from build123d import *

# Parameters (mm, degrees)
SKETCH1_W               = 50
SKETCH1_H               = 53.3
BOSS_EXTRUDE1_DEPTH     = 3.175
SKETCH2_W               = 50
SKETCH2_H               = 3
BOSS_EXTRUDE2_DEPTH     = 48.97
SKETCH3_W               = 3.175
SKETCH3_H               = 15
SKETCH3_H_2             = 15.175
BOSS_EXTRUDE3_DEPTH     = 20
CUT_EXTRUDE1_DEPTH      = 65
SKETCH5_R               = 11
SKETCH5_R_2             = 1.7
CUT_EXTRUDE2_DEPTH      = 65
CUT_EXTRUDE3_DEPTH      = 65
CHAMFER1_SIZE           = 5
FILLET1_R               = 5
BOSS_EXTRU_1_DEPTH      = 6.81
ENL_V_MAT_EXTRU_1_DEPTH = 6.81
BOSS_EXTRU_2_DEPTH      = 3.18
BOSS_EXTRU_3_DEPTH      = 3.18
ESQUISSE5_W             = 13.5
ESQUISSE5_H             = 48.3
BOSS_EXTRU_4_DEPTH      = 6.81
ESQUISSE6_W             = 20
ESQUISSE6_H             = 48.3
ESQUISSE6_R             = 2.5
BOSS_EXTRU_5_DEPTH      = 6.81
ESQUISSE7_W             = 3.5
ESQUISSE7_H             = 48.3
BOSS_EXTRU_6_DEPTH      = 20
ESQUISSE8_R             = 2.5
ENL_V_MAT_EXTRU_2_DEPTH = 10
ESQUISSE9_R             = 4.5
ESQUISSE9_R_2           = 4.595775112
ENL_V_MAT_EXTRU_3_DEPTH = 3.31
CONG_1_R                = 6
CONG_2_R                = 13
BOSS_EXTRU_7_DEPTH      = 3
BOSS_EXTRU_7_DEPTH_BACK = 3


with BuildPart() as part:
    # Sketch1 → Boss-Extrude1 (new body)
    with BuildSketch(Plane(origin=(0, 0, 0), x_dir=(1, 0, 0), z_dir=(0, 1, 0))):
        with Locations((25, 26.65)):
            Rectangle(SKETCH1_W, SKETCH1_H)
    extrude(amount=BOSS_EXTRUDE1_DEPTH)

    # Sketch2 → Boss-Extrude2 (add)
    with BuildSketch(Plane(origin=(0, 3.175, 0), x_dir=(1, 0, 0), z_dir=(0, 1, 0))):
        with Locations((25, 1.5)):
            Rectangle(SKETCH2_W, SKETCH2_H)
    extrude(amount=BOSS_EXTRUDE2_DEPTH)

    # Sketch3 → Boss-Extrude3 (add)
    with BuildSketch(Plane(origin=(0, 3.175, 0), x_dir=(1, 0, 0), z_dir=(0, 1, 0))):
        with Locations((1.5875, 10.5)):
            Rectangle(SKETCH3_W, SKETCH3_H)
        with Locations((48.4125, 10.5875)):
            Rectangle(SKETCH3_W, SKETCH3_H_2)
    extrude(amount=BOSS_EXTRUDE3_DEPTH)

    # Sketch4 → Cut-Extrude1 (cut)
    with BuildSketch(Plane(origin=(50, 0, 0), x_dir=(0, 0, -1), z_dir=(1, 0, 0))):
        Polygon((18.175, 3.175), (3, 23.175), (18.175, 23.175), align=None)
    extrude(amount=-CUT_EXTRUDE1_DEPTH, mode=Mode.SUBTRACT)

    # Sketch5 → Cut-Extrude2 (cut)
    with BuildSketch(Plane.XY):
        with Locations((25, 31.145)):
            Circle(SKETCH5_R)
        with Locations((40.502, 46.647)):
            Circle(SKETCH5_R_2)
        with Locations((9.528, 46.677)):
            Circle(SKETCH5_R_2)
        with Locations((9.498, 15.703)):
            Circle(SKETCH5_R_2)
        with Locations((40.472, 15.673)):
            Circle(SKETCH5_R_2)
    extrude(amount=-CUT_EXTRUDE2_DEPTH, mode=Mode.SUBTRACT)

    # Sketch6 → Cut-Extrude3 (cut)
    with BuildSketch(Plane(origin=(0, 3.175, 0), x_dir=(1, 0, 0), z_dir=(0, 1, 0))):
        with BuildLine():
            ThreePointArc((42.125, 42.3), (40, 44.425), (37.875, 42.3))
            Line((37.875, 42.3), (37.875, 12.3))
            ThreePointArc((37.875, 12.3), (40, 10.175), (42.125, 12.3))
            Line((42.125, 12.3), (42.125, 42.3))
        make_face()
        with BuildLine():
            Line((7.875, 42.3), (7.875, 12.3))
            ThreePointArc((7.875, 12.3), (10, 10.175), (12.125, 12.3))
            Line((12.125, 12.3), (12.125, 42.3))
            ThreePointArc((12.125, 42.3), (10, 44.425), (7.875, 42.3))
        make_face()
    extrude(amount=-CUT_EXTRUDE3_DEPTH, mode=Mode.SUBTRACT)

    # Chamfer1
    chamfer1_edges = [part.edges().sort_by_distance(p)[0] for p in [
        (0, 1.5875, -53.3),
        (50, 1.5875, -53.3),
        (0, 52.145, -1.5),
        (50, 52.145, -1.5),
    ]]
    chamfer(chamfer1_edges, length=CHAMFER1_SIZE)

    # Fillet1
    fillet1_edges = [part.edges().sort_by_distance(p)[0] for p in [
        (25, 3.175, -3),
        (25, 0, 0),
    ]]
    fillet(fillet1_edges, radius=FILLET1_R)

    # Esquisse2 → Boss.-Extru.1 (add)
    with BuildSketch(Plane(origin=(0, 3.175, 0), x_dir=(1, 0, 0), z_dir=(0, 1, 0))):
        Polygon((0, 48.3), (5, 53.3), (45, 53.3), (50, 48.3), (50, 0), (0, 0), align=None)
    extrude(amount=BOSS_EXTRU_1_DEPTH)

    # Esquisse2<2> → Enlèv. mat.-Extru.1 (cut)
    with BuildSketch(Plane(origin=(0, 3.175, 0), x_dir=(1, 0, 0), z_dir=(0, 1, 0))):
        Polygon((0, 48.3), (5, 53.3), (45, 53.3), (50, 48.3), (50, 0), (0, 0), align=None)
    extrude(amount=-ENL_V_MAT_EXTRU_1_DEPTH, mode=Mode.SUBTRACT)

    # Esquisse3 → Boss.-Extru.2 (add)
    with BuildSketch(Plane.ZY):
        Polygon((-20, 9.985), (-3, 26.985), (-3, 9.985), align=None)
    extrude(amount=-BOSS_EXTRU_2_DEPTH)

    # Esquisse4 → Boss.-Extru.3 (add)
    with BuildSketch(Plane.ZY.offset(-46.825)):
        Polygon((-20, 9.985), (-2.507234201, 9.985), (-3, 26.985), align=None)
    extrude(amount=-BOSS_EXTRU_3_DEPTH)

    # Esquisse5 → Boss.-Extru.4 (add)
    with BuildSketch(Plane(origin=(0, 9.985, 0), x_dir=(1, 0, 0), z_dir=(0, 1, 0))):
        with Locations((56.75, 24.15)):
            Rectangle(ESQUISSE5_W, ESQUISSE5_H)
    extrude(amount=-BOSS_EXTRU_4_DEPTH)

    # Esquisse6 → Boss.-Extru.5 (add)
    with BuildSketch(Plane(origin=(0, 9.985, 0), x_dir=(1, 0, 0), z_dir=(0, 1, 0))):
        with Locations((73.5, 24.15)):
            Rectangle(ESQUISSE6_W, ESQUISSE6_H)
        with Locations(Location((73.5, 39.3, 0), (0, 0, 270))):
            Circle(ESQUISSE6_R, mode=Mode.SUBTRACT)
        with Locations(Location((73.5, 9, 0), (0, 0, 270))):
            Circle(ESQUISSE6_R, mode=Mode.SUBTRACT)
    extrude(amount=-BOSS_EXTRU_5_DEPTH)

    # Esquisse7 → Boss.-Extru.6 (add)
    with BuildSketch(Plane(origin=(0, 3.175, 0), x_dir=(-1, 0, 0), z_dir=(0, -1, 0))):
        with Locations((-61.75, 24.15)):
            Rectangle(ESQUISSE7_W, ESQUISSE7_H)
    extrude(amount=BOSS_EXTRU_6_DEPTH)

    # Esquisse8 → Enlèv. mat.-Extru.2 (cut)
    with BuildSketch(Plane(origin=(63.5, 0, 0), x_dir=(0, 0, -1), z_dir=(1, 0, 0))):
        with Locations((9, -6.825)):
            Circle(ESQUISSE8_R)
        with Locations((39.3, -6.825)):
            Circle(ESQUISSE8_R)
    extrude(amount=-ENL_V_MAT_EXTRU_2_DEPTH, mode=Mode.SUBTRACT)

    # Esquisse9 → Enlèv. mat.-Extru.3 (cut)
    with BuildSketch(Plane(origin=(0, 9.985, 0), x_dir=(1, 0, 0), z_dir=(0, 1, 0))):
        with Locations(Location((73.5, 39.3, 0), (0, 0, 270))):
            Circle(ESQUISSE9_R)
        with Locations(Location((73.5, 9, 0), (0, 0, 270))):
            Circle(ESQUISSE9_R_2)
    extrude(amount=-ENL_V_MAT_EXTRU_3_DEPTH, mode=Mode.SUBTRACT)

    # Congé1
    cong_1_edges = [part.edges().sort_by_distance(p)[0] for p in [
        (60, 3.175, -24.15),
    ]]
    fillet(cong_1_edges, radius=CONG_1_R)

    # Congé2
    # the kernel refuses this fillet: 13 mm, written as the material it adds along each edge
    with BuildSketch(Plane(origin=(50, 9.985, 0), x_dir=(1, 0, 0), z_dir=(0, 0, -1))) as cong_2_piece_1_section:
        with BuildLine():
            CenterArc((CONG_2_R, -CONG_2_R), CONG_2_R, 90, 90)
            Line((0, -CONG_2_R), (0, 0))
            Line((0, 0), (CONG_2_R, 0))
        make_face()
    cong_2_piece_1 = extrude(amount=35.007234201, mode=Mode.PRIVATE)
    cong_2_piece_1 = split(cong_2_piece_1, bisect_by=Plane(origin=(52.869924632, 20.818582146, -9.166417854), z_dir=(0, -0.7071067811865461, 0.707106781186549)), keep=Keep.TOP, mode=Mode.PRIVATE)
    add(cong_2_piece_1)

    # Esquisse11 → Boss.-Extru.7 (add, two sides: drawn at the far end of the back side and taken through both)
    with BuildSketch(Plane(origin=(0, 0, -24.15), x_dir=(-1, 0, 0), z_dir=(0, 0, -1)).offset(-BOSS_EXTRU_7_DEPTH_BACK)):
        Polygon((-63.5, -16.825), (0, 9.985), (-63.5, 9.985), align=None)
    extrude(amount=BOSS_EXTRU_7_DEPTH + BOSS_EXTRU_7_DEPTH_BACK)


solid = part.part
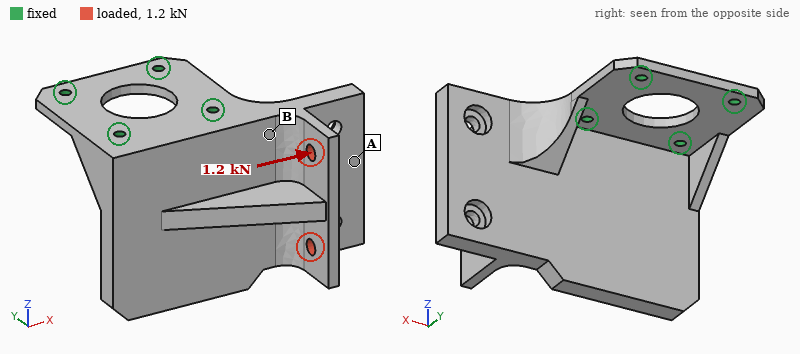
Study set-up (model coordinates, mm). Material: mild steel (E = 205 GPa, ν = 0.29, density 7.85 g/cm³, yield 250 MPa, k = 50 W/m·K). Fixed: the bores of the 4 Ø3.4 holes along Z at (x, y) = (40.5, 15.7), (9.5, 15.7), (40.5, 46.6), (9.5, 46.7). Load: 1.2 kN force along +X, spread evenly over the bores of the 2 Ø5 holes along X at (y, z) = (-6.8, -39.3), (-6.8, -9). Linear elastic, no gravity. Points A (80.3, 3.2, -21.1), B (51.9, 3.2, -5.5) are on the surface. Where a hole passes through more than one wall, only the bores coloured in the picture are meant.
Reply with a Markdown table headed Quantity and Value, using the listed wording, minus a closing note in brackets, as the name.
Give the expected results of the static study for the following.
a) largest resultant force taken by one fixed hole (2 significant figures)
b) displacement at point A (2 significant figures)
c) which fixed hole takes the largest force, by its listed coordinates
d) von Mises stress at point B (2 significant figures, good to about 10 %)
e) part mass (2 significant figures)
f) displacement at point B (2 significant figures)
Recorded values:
| Quantity | Value |
|---|---|
| largest resultant force taken by one fixed hole | 1.3 kN |
| displacement at point A | 20 µm |
| which fixed hole takes the largest force, by its listed coordinates | (9.5, 15.7) |
| von Mises stress at point B | 18 MPa |
| part mass | 320 g |
| displacement at point B | 7.9 µm |
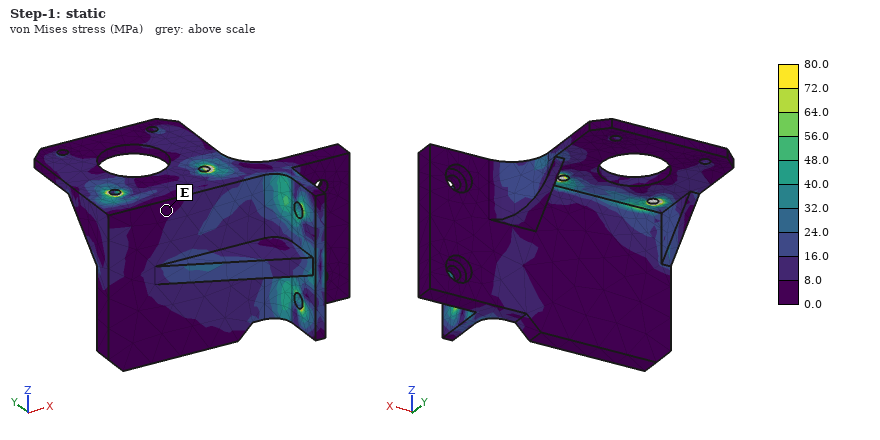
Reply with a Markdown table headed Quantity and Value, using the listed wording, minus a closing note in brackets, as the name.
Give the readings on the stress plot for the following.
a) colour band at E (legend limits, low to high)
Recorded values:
| Quantity | Value |
|---|---|
| colour band at E | 0.0 to 8.0 MPa |
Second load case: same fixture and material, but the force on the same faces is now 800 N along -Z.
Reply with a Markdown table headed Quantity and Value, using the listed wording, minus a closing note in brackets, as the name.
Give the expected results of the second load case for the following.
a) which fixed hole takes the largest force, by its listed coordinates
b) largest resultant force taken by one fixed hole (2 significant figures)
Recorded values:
| Quantity | Value |
|---|---|
| which fixed hole takes the largest force, by its listed coordinates | (40.5, 15.7) |
| largest resultant force taken by one fixed hole | 1.5 kN |
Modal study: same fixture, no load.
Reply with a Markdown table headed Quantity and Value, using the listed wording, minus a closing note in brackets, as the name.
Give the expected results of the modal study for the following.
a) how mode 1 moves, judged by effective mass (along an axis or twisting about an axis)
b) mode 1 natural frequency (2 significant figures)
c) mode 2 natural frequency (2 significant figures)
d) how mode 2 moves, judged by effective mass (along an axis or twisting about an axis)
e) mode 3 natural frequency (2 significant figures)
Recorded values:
| Quantity | Value |
|---|---|
| how mode 1 moves, judged by effective mass | along Y |
| mode 1 natural frequency | 900 Hz |
| mode 2 natural frequency | 2100 Hz |
| how mode 2 moves, judged by effective mass | along X |
| mode 3 natural frequency | 3000 Hz |
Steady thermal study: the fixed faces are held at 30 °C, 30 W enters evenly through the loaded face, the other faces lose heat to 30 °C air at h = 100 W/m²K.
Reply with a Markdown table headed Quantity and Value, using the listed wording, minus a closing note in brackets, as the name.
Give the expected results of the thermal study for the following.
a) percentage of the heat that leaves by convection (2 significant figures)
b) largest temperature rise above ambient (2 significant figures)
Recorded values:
| Quantity | Value |
|---|---|
| percentage of the heat that leaves by convection | 80 % |
| largest temperature rise above ambient | 61 K |
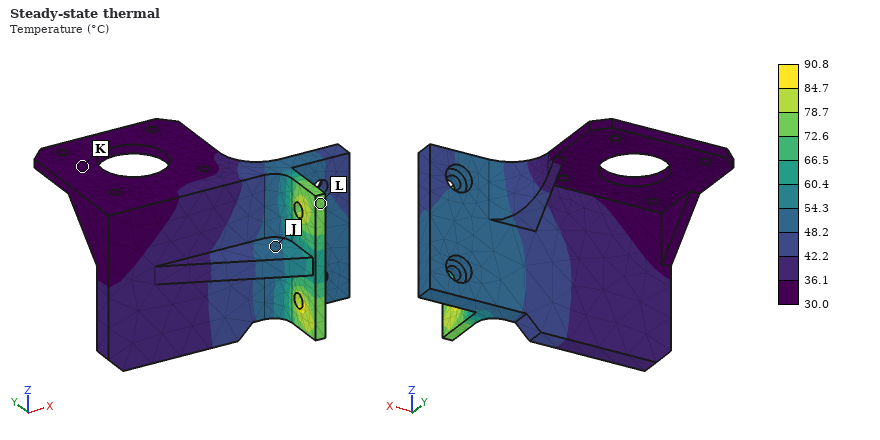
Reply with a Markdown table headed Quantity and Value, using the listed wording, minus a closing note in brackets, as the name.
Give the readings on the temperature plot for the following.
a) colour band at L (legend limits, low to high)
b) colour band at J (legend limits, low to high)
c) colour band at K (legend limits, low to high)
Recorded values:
| Quantity | Value |
|---|---|
| colour band at L | 72.6 to 78.7 °C |
| colour band at J | 48.2 to 54.3 °C |
| colour band at K | 30.0 to 36.1 °C |
